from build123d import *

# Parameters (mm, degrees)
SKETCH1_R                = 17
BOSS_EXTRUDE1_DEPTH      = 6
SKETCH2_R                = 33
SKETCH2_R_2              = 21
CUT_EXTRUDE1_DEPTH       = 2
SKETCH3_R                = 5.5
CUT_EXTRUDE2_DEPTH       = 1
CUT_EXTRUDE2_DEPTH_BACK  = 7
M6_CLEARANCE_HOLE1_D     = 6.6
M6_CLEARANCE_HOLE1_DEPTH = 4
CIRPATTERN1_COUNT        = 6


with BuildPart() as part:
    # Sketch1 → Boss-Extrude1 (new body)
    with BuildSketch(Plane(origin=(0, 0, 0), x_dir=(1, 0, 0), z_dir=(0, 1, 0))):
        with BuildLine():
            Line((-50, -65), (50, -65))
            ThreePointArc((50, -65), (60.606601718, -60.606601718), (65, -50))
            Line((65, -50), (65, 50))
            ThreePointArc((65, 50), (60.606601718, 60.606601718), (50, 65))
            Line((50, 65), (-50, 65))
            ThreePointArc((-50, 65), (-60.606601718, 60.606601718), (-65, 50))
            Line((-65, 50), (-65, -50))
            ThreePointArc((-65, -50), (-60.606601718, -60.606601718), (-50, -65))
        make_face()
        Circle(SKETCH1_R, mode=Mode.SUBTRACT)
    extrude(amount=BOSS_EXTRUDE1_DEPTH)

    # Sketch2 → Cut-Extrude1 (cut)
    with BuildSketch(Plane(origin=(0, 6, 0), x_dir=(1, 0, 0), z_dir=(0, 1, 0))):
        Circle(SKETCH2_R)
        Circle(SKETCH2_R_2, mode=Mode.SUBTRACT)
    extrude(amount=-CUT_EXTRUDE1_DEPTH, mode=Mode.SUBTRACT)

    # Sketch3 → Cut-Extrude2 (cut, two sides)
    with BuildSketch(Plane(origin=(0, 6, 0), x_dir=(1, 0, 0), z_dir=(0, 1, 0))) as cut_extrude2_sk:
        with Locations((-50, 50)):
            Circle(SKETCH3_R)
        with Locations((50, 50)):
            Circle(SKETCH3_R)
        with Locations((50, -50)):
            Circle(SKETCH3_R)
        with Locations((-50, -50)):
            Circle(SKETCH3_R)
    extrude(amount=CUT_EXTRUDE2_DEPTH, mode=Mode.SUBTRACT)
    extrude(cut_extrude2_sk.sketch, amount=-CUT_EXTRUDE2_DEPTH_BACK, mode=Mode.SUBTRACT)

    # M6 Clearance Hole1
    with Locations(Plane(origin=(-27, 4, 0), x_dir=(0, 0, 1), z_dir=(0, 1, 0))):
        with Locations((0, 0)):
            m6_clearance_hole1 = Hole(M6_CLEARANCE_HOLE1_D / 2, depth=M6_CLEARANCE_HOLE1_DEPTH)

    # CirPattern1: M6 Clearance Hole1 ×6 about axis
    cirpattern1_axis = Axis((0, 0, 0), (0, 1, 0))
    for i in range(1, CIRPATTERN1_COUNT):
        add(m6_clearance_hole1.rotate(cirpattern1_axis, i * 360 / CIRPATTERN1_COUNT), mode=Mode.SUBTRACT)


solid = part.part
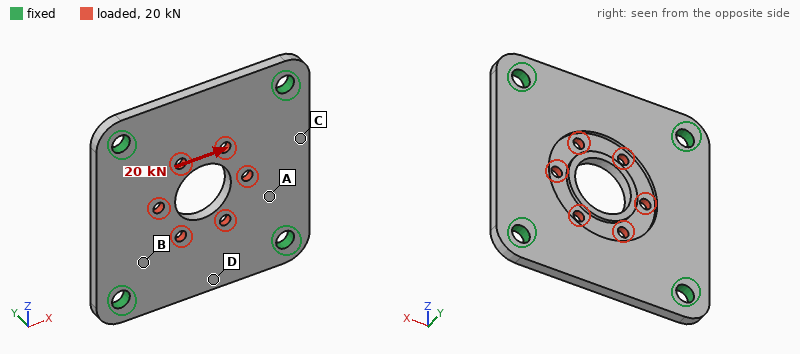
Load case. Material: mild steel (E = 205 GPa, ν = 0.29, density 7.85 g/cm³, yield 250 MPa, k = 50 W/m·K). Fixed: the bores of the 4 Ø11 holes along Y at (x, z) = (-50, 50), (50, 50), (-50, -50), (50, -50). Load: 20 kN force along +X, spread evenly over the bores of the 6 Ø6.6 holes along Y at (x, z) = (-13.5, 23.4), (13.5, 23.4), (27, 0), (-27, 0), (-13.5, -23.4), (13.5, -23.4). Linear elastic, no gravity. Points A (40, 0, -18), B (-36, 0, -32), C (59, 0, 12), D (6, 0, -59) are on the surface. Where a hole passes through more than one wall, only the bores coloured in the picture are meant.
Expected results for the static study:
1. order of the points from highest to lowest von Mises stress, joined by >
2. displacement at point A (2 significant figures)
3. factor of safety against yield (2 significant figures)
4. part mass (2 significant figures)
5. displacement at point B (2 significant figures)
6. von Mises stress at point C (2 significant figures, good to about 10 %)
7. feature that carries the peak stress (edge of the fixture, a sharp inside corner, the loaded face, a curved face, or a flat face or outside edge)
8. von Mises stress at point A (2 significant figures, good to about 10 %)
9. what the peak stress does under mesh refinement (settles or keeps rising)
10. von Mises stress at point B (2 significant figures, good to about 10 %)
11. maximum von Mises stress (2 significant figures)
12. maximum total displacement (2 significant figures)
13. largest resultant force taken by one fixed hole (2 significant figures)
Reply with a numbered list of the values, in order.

1. B > A > C > D
2. 6.9 µm
3. 2.5
4. 690 g
5. 4.4 µm
6. 12 MPa
7. the loaded face
8. 24 MPa
9. settles
10. 31 MPa
11. 98 MPa
12. 11 µm
13. 5.4 kN
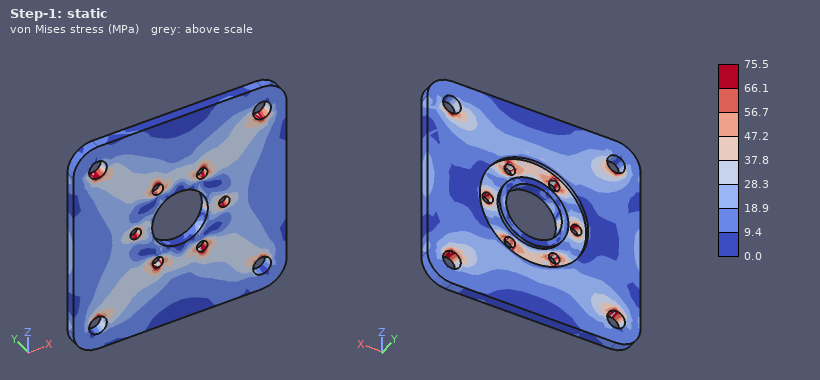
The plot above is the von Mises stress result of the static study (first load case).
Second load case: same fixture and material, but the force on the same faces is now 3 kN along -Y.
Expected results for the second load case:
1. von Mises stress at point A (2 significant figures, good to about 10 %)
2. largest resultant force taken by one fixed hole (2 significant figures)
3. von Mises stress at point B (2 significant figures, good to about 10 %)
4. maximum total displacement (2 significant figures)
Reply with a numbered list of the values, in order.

1. 29 MPa
2. 860 N
3. 23 MPa
4. 87 µm
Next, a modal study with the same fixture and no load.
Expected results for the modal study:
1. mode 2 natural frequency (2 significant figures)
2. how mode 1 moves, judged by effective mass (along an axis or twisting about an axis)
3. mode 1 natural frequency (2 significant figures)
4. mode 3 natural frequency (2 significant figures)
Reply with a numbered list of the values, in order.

1. 3600 Hz
2. along Y
3. 2500 Hz
4. 3600 Hz
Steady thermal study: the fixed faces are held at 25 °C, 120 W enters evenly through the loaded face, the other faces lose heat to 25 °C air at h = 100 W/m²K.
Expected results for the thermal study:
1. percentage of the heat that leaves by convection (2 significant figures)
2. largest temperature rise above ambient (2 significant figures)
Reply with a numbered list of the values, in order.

1. 63 %
2. 67 K
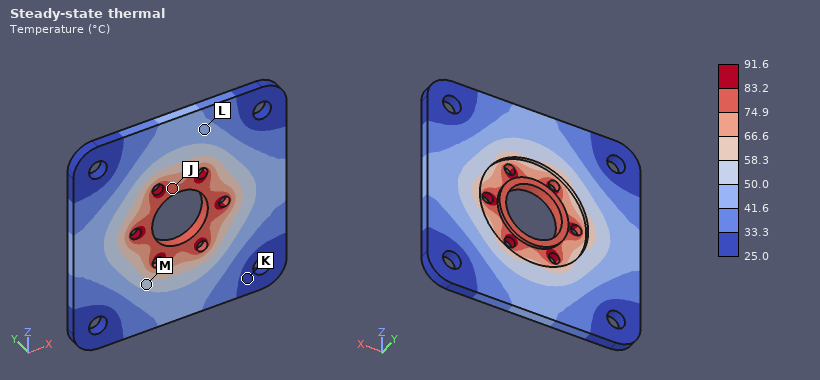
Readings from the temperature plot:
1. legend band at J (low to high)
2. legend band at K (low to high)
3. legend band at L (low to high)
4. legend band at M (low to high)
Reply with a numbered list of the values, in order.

1. 74.9 to 83.2 °C
2. 25.0 to 33.3 °C
3. 41.6 to 50.0 °C
4. 50.0 to 58.3 °C
